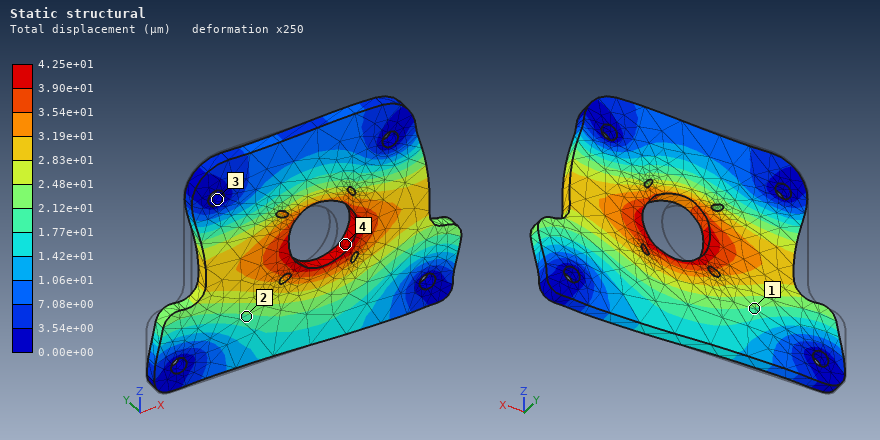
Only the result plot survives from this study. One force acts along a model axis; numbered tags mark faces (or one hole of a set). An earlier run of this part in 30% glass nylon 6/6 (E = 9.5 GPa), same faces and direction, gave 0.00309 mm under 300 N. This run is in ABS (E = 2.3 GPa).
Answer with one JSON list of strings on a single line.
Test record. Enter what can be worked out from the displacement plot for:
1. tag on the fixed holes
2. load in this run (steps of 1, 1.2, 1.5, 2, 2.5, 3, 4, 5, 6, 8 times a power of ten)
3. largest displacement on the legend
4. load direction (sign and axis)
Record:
["3", "1 kN", "4.25e+01 µm", "+X"]
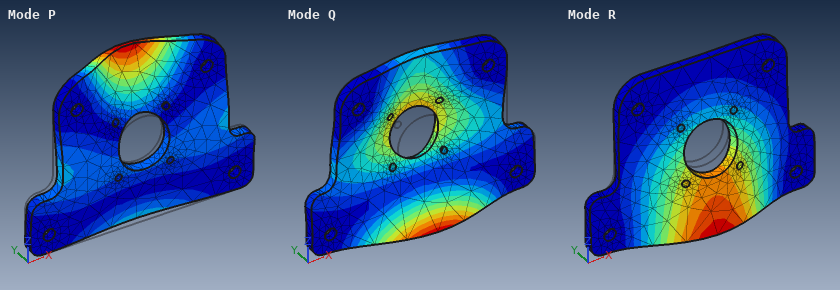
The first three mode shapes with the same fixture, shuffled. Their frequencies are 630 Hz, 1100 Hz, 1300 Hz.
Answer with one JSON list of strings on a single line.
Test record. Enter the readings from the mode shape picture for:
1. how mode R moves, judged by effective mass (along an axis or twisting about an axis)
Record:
["along Y"]
